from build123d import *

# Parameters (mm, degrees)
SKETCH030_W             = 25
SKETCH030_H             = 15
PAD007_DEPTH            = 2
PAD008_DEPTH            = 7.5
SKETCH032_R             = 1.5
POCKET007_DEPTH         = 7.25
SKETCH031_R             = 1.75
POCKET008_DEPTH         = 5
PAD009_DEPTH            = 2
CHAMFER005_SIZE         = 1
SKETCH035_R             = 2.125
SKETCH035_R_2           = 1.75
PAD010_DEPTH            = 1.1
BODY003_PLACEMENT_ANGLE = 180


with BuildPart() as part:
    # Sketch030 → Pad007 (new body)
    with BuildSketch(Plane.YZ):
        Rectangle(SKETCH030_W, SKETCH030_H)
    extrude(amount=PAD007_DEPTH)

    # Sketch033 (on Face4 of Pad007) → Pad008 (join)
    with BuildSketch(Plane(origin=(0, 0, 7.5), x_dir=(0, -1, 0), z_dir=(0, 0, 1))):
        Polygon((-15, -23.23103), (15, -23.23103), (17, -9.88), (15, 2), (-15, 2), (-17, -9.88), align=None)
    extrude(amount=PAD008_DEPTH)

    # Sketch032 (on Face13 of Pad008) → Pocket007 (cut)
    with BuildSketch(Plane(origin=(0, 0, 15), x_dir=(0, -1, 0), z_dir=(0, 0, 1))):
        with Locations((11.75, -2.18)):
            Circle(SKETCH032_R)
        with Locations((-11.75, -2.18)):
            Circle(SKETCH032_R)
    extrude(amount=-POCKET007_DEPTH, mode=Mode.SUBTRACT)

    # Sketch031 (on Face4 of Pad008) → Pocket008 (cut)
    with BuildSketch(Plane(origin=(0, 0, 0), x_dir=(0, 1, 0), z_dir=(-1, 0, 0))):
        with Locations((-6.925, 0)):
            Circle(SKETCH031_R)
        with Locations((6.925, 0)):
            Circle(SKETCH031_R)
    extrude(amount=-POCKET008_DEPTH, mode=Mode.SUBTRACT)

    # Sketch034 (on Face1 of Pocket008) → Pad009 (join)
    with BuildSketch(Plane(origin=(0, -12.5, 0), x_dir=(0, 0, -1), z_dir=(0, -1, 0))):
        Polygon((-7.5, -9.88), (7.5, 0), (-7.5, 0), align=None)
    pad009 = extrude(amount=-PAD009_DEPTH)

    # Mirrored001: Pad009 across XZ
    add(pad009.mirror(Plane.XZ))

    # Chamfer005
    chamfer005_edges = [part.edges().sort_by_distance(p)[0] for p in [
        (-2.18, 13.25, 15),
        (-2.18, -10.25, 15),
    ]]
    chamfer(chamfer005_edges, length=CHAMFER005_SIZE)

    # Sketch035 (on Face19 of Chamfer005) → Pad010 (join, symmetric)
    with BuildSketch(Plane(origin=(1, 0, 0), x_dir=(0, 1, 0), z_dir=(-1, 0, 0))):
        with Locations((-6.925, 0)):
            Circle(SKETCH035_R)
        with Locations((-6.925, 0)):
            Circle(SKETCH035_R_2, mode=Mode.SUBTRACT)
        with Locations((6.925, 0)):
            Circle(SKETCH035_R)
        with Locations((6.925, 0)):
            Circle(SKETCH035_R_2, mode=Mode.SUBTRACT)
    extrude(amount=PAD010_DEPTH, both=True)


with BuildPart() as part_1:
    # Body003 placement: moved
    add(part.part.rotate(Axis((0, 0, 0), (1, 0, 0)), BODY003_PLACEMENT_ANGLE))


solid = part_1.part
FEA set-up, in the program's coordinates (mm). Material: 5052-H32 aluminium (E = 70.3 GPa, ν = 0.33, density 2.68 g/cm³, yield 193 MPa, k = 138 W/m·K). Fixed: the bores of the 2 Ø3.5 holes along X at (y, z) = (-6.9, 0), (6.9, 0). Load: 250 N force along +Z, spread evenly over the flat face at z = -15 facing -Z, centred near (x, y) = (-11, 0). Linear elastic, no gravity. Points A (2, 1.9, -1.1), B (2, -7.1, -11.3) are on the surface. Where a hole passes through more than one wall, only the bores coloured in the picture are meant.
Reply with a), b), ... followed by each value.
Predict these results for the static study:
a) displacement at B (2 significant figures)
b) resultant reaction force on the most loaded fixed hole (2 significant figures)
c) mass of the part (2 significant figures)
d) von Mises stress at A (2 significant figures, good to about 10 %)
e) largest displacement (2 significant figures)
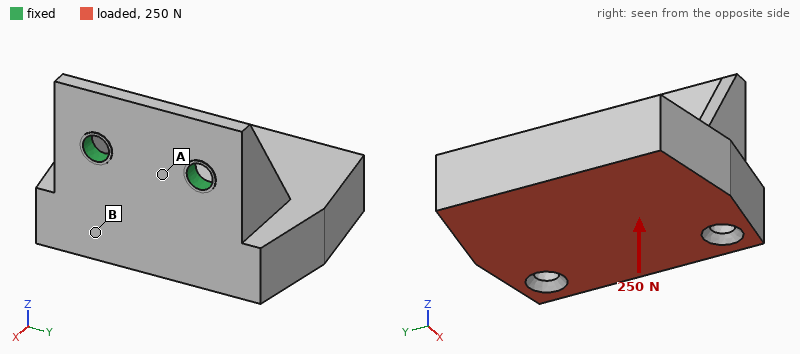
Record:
a) 0.035 mm
b) 130 N
c) 19 g
d) 32 MPa
e) 0.11 mm
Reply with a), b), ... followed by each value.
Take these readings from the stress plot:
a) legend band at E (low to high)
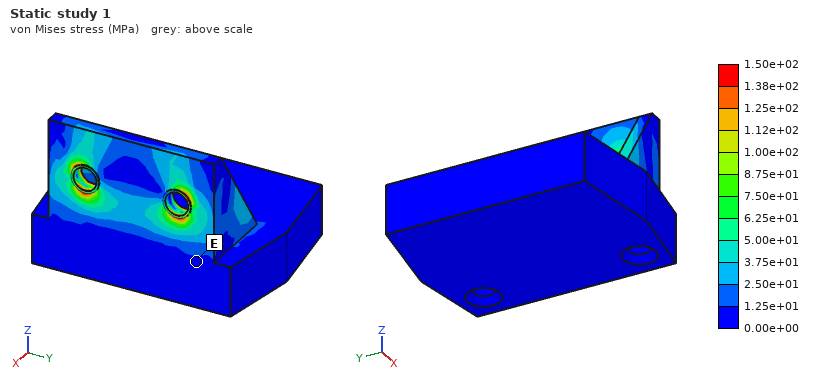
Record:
a) 0.00e+00 to 1.25e+01 MPa
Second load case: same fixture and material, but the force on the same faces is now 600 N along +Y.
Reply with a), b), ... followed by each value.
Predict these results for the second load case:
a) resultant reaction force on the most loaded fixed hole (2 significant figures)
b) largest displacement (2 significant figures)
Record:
a) 710 N
b) 55 µm
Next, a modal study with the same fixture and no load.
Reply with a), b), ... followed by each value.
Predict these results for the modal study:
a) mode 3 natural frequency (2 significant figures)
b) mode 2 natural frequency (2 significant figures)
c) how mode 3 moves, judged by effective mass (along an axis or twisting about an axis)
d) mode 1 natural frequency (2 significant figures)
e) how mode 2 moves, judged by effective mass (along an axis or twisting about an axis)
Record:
a) 11 kHz
b) 4400 Hz
c) along X
d) 2100 Hz
e) along Y
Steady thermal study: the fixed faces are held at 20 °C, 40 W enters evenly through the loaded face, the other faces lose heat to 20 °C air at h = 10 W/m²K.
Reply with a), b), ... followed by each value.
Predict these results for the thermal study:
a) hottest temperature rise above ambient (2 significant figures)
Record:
a) 52 K
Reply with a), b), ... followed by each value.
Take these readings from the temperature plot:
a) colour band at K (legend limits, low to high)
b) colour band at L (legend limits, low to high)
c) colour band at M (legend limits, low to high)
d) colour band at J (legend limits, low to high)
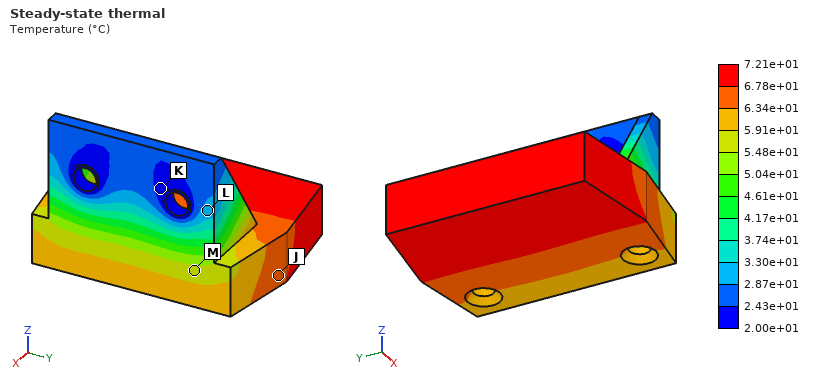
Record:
a) 2.00e+01 to 2.43e+01 °C
b) 2.87e+01 to 3.30e+01 °C
c) 5.48e+01 to 5.91e+01 °C
d) 6.34e+01 to 6.78e+01 °C
